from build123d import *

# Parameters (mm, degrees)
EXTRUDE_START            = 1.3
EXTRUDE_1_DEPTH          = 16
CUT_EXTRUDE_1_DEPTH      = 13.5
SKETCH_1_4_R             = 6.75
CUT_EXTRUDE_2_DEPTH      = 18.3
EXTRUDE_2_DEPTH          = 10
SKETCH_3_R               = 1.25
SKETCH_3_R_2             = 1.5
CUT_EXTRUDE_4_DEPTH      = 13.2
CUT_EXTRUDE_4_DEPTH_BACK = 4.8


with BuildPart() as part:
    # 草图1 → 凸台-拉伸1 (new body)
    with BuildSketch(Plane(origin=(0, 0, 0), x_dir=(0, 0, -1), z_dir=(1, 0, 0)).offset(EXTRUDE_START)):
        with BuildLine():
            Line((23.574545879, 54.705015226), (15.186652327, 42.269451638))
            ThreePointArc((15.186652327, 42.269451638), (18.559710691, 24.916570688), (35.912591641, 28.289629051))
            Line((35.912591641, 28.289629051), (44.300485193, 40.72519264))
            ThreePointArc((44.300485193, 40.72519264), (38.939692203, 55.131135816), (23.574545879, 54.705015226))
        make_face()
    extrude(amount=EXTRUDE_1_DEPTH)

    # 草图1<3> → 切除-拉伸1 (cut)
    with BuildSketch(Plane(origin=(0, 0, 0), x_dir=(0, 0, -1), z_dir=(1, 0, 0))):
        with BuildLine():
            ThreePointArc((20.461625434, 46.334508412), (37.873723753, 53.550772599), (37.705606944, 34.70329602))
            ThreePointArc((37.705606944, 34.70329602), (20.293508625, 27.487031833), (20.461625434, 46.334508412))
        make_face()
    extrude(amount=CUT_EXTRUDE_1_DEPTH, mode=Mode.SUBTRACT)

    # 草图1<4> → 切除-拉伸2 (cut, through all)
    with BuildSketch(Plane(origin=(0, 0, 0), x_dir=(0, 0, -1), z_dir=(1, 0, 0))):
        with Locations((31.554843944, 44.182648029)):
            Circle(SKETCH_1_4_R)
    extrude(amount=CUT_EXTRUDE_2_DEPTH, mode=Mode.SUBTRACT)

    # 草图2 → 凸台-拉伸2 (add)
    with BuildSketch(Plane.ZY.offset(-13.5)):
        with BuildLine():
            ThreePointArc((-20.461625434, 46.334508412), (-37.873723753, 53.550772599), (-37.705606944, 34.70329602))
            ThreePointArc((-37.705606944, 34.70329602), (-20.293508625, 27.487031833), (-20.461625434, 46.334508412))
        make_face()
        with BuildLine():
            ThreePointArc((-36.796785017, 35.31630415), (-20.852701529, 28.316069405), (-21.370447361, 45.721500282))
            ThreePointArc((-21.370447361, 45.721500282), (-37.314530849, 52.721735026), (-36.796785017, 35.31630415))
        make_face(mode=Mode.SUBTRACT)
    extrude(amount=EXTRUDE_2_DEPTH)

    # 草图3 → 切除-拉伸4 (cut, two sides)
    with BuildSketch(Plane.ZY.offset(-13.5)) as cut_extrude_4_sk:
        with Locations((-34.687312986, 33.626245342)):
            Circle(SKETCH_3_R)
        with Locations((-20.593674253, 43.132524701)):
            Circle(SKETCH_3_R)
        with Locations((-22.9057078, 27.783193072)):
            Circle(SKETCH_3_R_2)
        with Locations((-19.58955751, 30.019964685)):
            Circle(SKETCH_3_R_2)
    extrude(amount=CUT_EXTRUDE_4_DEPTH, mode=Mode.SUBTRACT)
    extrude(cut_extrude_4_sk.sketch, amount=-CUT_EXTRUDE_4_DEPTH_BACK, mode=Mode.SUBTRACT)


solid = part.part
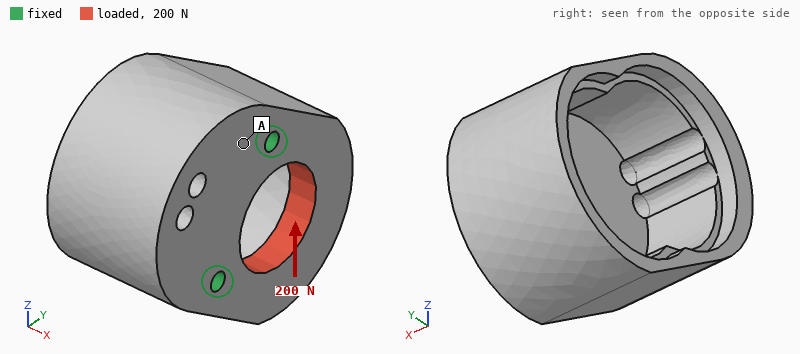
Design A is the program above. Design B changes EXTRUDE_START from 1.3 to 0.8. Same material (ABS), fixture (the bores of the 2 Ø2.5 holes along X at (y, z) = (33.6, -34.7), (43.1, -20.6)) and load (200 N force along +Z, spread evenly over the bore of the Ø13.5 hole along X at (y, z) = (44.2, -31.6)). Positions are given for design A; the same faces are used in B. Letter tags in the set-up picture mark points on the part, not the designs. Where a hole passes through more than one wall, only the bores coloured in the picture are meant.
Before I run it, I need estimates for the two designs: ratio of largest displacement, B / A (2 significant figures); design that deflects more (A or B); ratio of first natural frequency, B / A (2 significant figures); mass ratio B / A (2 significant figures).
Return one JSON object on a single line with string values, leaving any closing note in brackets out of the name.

{"ratio of largest displacement, B / A": "1.1", "design that deflects more": "B", "ratio of first natural frequency, B / A": "0.88", "mass ratio B / A": "0.96"}
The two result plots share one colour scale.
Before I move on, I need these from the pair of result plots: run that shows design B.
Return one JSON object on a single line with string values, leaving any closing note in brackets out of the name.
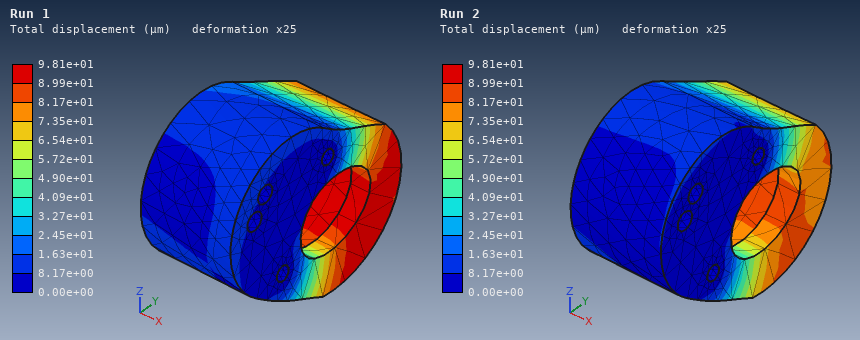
{"run that shows design B": "Run 1"}
